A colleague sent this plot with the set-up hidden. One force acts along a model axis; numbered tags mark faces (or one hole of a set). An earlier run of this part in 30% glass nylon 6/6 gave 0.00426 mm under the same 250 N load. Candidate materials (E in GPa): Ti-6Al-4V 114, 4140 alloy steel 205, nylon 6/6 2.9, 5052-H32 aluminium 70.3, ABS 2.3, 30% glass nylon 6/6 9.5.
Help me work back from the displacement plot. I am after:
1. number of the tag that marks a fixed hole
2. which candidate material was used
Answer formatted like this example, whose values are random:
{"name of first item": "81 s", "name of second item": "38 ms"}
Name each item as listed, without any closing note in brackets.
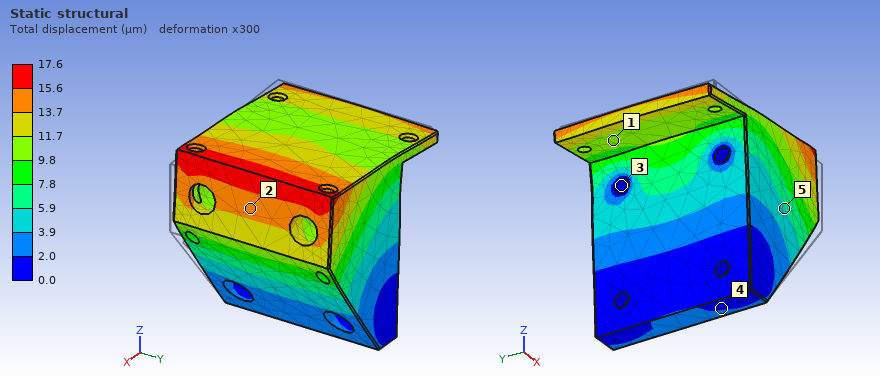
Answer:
{"number of the tag that marks a fixed hole": "3", "which candidate material was used": "ABS"}
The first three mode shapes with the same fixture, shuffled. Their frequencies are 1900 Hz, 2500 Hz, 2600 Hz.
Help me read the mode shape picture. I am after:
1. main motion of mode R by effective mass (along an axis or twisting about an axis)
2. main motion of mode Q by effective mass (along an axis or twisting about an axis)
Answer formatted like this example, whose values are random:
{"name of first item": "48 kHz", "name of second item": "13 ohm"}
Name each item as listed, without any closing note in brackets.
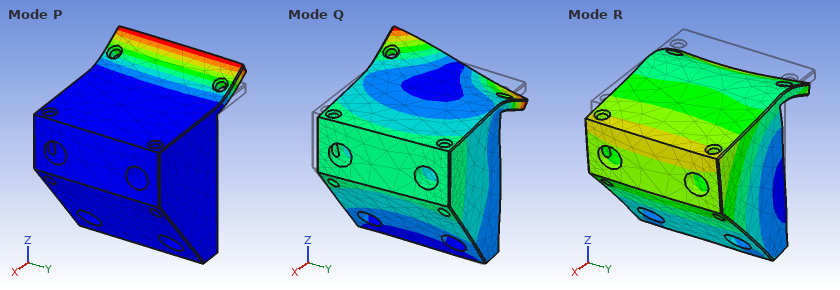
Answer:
{"main motion of mode R by effective mass": "along Z", "main motion of mode Q by effective mass": "along Y"}
